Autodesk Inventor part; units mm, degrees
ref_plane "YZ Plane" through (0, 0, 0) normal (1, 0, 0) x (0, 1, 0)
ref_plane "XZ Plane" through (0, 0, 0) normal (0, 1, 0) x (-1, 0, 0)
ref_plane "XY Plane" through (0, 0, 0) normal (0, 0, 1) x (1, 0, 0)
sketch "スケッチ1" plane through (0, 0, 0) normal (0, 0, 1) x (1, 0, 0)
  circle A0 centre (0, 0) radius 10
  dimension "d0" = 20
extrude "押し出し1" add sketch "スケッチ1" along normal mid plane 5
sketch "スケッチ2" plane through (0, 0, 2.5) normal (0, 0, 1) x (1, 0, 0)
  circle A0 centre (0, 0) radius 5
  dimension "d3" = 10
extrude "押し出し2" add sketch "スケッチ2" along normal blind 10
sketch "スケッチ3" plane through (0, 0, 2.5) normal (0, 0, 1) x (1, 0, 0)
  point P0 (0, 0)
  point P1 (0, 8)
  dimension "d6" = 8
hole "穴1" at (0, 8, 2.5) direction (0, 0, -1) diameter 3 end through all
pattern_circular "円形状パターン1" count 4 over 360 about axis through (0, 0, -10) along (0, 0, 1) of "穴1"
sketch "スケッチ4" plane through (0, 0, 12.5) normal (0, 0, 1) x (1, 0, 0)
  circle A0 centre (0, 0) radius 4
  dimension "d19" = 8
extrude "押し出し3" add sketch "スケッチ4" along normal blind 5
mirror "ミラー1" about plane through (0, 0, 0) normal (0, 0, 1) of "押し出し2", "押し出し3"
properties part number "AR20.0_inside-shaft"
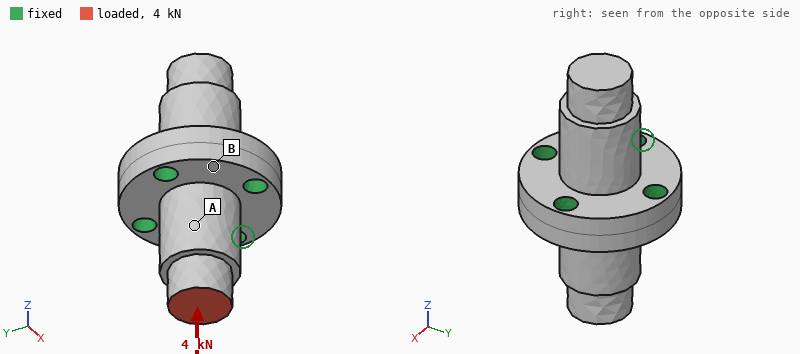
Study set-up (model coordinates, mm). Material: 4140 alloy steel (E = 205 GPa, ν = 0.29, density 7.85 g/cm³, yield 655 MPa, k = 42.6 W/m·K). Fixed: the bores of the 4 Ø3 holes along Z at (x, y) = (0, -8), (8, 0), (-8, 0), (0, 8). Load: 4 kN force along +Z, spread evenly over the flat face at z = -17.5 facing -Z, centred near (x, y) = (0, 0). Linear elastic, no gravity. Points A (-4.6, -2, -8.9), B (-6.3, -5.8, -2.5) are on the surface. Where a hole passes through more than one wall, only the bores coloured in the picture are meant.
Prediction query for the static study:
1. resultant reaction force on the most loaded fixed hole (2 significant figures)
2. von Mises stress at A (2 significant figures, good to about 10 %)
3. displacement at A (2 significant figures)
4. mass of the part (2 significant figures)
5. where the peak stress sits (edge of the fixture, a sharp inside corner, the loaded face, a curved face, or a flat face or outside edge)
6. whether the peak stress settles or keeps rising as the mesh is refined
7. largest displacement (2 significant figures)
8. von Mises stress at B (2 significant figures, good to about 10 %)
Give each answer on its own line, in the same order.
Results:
1.0 kN
47 MPa
3.2 µm
27 g
edge of the fixture
keeps rising
6.2 µm
14 MPa
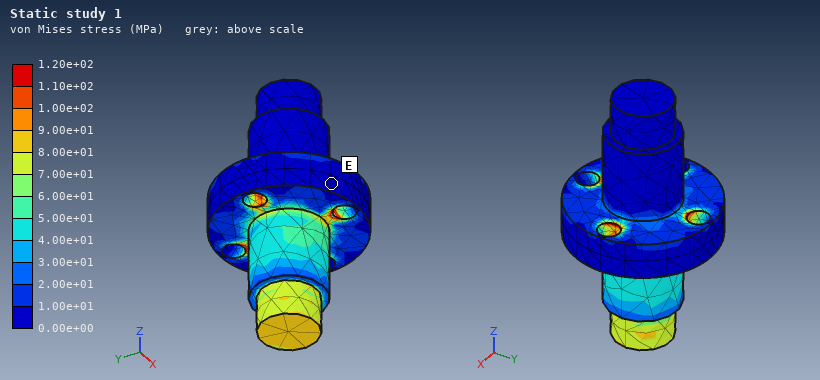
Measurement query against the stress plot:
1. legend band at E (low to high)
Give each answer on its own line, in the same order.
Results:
0.00e+00 to 1.00e+01 MPa
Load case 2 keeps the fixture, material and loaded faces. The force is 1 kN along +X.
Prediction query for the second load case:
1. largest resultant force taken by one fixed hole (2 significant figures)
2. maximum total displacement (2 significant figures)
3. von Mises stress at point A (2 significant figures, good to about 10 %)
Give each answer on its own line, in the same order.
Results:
1.2 kN
23 µm
80 MPa
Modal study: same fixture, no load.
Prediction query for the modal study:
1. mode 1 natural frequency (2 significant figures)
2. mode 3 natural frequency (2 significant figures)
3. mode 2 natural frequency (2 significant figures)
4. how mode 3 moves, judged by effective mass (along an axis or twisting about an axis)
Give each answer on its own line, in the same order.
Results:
22 kHz
26 kHz
22 kHz
along X
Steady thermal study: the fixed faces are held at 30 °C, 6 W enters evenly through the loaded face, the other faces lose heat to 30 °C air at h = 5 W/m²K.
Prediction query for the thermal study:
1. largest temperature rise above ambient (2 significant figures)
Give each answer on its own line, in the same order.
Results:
38 K
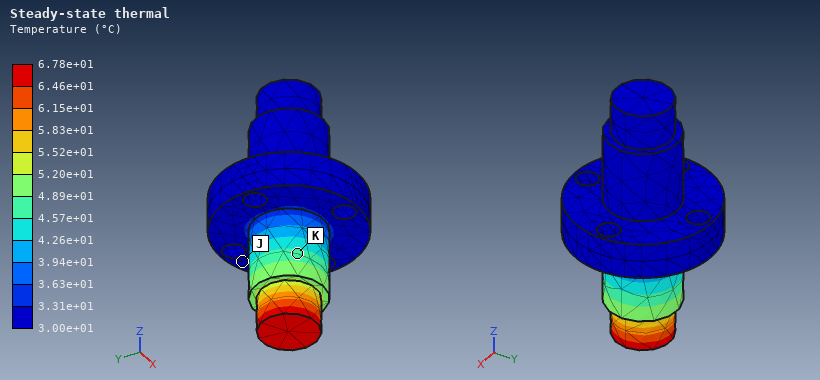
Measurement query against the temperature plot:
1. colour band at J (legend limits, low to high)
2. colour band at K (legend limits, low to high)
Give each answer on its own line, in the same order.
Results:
3.00e+01 to 3.31e+01 °C
4.57e+01 to 4.89e+01 °C
